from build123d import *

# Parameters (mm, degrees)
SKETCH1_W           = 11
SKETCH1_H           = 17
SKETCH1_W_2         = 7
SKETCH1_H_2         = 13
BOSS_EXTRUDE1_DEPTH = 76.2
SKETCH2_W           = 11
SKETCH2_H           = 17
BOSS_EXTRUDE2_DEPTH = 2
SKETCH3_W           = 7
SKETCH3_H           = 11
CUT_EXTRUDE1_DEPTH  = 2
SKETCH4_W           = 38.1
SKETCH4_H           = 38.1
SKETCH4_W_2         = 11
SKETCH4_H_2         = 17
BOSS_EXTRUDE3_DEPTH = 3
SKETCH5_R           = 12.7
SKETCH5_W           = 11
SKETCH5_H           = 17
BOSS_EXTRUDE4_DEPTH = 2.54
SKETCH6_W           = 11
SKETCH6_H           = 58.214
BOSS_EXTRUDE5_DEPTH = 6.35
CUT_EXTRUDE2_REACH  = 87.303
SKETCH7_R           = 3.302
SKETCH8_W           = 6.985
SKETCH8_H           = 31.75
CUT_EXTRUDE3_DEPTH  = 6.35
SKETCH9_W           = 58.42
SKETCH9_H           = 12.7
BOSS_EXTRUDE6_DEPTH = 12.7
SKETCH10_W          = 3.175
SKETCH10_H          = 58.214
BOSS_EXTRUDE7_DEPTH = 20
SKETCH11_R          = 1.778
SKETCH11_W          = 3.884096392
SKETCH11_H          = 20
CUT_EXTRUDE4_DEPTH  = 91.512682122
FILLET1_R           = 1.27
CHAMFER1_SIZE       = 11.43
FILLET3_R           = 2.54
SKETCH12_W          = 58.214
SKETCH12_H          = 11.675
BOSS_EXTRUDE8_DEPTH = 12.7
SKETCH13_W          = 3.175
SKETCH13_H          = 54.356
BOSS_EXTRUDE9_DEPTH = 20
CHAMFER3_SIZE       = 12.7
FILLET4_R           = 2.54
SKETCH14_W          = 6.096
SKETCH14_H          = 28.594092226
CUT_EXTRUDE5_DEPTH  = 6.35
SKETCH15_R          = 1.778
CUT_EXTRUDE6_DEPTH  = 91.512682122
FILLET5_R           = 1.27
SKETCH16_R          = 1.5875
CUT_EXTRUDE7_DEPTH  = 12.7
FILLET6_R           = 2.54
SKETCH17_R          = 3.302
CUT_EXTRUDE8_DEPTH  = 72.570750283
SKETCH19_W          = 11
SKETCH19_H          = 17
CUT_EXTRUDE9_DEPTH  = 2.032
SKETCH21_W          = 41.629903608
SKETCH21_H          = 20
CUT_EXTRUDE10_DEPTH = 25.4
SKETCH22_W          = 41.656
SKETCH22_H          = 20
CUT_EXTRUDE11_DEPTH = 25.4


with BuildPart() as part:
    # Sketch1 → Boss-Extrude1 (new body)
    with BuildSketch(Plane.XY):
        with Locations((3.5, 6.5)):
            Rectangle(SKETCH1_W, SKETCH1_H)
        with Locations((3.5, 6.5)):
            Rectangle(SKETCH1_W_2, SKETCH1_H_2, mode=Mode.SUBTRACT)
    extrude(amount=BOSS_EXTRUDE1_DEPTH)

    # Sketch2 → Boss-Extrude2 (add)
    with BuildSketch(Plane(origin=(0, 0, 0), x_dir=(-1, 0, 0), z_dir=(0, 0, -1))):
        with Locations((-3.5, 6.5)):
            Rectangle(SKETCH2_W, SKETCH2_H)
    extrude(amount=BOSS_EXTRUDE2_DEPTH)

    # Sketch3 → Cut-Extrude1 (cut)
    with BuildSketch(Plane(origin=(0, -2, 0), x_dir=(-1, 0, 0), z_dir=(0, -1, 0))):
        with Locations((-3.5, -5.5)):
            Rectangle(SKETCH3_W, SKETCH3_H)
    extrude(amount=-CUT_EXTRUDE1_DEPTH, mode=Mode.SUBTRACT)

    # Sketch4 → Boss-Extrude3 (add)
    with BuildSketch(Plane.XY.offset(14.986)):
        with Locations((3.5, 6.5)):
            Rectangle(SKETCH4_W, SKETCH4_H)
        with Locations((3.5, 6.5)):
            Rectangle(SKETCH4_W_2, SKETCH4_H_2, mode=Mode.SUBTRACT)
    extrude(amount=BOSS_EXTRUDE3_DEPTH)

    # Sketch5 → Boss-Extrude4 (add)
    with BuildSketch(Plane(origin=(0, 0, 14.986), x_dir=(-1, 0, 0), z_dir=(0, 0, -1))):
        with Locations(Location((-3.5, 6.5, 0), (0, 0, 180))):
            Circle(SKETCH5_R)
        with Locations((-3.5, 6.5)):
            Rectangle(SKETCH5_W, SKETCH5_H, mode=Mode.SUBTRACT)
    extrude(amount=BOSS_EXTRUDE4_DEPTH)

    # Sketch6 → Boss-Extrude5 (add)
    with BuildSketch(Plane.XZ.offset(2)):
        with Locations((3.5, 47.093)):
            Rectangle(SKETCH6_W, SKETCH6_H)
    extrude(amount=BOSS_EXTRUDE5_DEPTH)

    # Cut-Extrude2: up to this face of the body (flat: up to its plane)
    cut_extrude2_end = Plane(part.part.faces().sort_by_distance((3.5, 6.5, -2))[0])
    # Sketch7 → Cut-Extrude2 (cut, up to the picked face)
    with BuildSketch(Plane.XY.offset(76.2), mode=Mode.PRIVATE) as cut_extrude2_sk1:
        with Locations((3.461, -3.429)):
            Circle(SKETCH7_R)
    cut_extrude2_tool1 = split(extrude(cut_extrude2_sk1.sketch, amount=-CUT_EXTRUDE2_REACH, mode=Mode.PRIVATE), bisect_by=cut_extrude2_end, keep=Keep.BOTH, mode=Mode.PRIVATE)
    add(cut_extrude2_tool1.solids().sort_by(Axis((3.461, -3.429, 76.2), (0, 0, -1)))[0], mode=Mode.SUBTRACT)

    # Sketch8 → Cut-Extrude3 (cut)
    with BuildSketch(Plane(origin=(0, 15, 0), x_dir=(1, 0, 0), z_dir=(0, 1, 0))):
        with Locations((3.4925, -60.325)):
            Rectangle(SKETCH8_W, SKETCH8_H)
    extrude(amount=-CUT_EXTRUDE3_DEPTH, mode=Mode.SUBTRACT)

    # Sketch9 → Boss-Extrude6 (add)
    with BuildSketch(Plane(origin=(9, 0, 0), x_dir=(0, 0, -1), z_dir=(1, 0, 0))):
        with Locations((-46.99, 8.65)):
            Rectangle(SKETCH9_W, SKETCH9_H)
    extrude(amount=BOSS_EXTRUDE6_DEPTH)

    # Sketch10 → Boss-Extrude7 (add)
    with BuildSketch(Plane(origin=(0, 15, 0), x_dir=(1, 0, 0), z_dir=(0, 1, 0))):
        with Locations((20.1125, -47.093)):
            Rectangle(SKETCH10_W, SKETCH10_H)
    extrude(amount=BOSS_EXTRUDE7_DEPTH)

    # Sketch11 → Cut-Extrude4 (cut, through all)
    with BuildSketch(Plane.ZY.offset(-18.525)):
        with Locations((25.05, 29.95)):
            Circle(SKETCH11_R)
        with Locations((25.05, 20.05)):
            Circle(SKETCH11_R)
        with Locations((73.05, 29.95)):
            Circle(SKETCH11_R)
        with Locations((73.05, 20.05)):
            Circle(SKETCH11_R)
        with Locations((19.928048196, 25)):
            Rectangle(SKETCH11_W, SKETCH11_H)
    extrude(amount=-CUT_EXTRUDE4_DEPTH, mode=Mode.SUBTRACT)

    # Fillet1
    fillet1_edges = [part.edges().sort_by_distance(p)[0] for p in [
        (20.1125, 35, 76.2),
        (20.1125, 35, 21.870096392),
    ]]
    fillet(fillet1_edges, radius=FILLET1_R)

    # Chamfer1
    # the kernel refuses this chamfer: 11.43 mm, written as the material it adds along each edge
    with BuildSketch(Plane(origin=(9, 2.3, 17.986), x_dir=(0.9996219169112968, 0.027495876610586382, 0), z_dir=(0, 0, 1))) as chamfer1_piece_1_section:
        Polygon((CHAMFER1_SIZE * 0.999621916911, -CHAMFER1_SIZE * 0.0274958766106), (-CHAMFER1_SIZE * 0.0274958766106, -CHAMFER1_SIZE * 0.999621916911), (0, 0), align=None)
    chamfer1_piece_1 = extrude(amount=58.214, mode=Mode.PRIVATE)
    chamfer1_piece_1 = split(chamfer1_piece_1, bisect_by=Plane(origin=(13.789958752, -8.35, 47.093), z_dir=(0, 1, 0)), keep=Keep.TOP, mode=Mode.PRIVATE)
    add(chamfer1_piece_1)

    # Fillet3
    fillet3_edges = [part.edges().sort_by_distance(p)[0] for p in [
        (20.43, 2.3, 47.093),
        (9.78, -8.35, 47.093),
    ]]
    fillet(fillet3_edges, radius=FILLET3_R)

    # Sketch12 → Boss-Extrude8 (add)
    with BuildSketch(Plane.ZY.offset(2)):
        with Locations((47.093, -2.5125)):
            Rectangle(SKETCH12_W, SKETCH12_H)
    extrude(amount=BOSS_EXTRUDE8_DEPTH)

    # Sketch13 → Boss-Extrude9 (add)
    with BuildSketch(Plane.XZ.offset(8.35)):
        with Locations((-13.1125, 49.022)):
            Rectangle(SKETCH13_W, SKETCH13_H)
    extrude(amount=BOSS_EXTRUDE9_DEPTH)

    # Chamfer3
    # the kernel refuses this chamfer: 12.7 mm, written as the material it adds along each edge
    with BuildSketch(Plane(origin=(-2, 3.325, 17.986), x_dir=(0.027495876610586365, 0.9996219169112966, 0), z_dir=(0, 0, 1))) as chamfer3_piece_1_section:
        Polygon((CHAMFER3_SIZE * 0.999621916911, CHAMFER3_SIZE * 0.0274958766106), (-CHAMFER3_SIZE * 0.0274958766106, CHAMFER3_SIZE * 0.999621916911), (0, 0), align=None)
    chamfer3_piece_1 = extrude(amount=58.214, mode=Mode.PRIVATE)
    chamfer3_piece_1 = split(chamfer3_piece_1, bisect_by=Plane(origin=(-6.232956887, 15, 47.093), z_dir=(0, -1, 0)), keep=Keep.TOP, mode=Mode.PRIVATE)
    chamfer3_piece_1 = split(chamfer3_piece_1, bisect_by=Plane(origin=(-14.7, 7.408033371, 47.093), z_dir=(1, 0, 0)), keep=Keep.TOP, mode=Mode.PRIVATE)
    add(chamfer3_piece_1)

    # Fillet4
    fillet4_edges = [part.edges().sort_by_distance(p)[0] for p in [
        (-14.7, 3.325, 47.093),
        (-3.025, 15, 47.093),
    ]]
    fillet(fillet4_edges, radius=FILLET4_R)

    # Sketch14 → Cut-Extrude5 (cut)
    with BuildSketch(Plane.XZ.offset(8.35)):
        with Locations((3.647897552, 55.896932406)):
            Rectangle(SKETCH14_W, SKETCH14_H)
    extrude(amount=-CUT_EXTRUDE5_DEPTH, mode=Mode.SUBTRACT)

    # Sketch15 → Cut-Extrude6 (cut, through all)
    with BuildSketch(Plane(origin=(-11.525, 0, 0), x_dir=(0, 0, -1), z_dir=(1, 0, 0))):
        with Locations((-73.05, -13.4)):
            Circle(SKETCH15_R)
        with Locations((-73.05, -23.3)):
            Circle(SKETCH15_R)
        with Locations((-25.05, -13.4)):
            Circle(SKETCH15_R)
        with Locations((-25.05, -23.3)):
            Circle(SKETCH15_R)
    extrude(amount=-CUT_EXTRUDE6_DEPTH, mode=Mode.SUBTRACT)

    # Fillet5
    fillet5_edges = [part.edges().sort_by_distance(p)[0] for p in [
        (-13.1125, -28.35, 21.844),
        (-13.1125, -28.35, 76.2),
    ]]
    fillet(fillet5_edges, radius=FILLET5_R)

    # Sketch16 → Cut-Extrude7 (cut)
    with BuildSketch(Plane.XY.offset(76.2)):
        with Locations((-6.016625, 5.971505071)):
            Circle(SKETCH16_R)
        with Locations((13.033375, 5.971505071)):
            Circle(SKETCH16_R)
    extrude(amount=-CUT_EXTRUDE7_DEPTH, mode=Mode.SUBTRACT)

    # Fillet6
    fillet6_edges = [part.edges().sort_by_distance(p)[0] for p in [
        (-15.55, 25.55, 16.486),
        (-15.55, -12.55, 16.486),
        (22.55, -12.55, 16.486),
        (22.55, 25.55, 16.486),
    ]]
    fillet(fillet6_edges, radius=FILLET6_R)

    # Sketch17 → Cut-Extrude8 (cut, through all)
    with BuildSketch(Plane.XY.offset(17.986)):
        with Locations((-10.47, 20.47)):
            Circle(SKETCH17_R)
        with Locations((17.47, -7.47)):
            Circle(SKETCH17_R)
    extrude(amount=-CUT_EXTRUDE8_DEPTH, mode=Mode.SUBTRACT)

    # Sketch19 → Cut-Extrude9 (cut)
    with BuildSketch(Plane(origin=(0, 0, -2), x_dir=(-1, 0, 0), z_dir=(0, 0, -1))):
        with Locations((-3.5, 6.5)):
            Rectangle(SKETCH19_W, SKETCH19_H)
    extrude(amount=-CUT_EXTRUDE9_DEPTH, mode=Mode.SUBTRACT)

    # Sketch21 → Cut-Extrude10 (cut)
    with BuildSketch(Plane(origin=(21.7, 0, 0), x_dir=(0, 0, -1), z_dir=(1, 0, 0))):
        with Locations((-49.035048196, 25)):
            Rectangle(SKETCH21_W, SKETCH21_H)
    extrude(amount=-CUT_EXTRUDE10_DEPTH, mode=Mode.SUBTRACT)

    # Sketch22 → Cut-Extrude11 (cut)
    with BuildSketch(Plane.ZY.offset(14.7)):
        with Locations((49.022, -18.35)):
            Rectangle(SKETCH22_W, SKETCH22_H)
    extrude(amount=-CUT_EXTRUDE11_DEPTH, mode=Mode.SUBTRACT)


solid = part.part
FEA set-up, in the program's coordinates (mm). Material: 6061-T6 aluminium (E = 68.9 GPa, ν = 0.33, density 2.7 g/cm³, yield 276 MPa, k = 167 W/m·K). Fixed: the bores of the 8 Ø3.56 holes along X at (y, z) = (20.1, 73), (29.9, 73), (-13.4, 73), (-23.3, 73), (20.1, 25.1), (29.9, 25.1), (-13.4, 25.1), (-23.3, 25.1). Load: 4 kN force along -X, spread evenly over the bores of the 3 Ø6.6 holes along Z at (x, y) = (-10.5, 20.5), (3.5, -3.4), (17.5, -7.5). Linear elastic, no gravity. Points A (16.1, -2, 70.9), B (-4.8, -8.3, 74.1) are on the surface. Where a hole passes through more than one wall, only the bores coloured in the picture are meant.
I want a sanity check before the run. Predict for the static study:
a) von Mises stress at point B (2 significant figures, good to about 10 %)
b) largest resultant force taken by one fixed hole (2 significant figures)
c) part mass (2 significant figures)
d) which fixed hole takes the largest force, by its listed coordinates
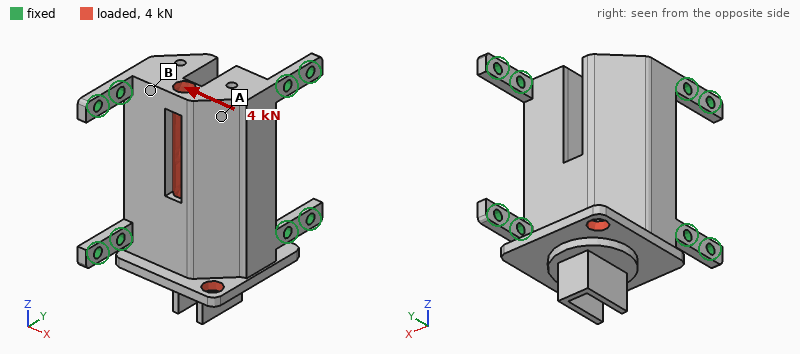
29 MPa
1.5 kN
110 g
(-13.4, 25.1)
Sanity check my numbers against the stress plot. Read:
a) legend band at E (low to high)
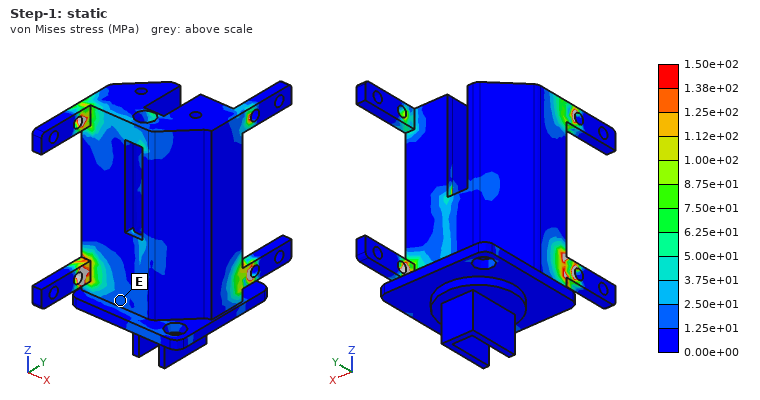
1.25e+01 to 2.50e+01 MPa
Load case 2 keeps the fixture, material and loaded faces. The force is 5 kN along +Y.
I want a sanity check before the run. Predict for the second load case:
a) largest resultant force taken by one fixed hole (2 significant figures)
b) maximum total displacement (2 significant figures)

1.7 kN
36 µm
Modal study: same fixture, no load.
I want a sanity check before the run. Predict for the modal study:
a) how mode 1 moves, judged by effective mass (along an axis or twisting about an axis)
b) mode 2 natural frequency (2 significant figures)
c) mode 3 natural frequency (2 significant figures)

along X
7000 Hz
7100 Hz
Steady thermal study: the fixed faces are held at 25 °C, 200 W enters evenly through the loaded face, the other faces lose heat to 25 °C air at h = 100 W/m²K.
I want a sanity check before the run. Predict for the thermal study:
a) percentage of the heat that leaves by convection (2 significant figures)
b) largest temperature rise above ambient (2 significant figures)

40 %
81 K
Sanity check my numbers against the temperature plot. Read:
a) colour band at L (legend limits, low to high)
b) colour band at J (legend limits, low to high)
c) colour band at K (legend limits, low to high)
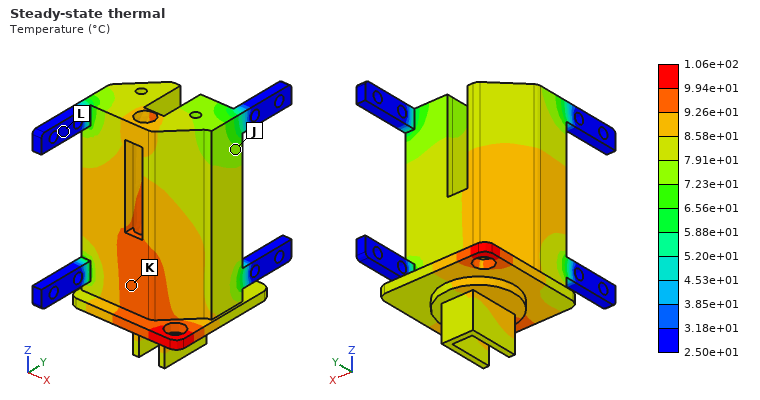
2.50e+01 to 3.18e+01 °C
7.23e+01 to 7.91e+01 °C
9.26e+01 to 9.94e+01 °C
